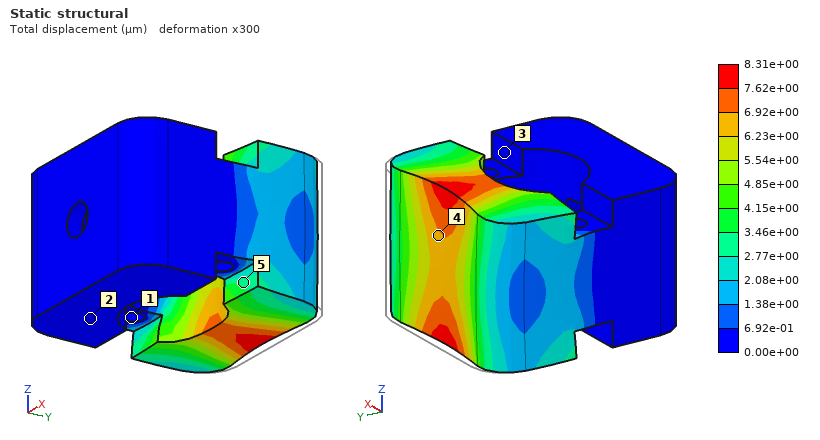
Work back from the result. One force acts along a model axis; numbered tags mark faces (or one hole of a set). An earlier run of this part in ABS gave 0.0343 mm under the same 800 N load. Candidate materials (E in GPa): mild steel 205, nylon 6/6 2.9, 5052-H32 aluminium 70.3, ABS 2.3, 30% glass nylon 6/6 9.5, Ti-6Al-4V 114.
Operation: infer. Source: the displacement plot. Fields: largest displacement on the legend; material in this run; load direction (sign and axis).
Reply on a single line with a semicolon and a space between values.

8.31e+00 µm; 30% glass nylon 6/6; -Y
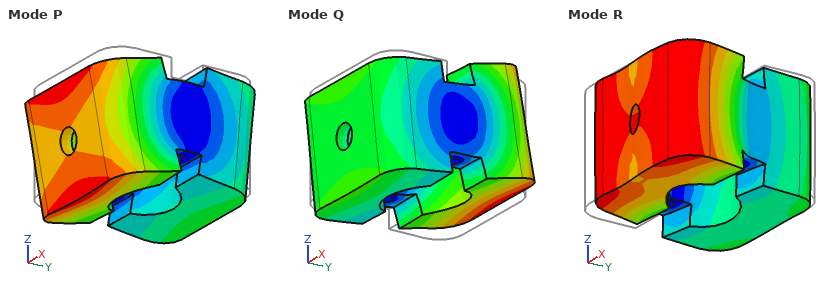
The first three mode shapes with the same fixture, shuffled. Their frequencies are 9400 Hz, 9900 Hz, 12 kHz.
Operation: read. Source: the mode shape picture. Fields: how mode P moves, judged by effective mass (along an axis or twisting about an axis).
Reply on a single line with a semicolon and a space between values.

along Z
